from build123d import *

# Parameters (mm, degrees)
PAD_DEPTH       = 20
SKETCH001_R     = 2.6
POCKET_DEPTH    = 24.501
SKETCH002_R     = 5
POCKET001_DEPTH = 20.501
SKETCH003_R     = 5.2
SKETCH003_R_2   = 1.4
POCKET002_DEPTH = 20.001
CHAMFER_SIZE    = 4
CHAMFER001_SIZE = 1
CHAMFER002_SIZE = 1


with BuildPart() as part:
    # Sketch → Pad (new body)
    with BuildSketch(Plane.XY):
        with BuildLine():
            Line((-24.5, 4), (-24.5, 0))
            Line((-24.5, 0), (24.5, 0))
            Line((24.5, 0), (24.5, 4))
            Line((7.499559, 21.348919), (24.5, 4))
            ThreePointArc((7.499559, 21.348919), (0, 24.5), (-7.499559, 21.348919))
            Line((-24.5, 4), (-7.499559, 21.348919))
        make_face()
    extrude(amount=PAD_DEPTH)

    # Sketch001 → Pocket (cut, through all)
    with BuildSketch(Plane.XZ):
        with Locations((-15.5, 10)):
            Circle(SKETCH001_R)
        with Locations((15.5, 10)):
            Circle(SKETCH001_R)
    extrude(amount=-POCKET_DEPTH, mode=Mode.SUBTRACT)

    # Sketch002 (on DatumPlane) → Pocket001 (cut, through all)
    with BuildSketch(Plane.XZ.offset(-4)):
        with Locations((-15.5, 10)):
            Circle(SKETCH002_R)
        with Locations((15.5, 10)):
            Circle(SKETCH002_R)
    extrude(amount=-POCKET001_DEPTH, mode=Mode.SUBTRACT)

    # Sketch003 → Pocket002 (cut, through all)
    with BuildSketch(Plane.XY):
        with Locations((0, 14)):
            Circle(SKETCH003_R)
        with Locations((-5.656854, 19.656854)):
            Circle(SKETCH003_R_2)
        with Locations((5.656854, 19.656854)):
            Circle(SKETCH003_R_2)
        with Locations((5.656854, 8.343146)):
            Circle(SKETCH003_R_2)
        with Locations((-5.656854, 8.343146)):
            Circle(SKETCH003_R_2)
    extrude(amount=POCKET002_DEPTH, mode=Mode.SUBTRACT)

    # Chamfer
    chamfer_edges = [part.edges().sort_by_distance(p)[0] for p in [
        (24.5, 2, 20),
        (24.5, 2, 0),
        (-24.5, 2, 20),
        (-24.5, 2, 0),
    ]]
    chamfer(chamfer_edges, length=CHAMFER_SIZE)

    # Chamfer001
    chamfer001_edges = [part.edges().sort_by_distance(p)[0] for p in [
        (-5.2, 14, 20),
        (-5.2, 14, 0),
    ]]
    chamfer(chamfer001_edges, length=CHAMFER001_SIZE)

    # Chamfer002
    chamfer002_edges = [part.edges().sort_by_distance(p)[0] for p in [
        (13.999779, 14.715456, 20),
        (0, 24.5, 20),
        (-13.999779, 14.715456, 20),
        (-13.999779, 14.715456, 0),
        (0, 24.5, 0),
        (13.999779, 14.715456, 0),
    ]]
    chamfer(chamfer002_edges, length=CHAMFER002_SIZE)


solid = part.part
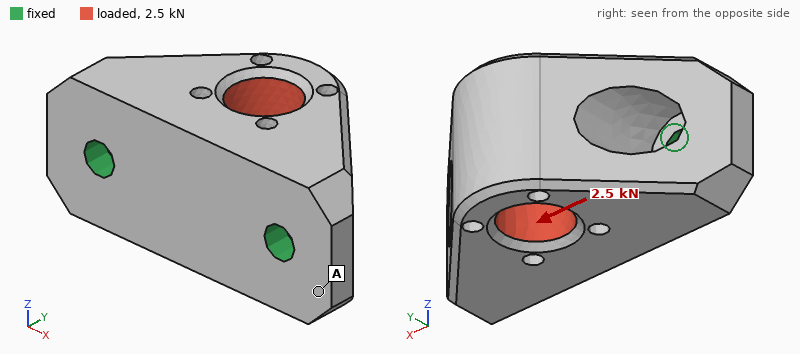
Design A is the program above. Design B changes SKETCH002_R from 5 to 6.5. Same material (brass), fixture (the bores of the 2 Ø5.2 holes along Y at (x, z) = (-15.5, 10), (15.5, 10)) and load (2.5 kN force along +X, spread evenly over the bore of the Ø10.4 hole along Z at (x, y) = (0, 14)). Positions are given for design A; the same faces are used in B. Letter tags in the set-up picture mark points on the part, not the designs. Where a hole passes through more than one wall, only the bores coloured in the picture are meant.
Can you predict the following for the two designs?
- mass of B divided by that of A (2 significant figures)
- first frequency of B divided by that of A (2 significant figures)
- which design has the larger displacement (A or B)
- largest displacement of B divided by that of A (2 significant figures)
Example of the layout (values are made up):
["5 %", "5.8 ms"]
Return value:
["0.91", "0.95", "B", "1.3"]
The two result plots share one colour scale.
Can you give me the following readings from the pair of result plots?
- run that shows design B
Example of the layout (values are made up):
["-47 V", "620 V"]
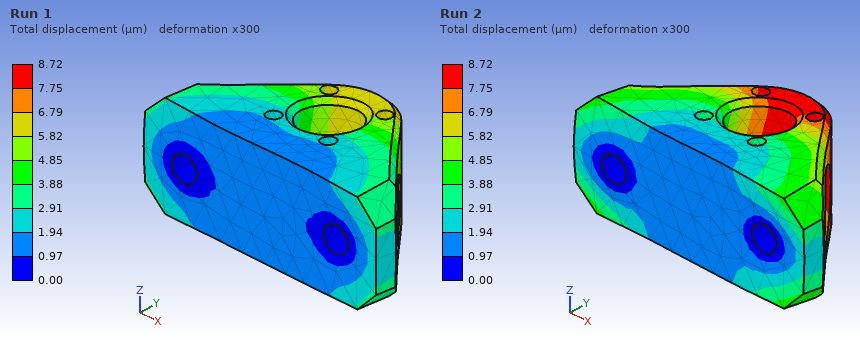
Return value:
["Run 2"]
